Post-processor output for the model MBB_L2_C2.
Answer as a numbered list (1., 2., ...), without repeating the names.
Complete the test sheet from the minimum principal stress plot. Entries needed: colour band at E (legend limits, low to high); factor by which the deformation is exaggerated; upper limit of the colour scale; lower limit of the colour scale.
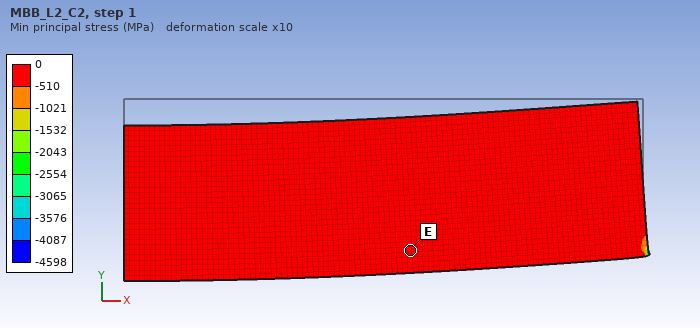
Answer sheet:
1. -510 to 0 MPa
2. 10
3. 0 MPa
4. -4598 MPa
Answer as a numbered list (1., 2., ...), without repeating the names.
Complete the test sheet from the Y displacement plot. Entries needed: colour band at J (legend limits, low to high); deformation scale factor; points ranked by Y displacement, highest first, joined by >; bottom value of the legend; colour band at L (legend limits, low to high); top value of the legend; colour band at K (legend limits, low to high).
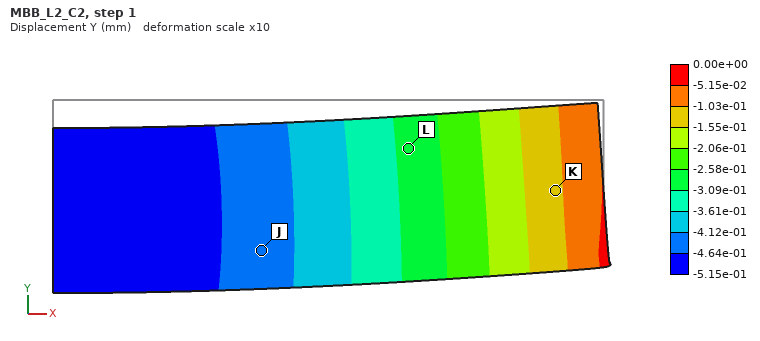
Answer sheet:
1. -4.64e-01 to -4.12e-01 mm
2. 10
3. K > L > J
4. -5.15e-01 mm
5. -3.09e-01 to -2.58e-01 mm
6. 0.00e+00 mm
7. -1.55e-01 to -1.03e-01 mm
